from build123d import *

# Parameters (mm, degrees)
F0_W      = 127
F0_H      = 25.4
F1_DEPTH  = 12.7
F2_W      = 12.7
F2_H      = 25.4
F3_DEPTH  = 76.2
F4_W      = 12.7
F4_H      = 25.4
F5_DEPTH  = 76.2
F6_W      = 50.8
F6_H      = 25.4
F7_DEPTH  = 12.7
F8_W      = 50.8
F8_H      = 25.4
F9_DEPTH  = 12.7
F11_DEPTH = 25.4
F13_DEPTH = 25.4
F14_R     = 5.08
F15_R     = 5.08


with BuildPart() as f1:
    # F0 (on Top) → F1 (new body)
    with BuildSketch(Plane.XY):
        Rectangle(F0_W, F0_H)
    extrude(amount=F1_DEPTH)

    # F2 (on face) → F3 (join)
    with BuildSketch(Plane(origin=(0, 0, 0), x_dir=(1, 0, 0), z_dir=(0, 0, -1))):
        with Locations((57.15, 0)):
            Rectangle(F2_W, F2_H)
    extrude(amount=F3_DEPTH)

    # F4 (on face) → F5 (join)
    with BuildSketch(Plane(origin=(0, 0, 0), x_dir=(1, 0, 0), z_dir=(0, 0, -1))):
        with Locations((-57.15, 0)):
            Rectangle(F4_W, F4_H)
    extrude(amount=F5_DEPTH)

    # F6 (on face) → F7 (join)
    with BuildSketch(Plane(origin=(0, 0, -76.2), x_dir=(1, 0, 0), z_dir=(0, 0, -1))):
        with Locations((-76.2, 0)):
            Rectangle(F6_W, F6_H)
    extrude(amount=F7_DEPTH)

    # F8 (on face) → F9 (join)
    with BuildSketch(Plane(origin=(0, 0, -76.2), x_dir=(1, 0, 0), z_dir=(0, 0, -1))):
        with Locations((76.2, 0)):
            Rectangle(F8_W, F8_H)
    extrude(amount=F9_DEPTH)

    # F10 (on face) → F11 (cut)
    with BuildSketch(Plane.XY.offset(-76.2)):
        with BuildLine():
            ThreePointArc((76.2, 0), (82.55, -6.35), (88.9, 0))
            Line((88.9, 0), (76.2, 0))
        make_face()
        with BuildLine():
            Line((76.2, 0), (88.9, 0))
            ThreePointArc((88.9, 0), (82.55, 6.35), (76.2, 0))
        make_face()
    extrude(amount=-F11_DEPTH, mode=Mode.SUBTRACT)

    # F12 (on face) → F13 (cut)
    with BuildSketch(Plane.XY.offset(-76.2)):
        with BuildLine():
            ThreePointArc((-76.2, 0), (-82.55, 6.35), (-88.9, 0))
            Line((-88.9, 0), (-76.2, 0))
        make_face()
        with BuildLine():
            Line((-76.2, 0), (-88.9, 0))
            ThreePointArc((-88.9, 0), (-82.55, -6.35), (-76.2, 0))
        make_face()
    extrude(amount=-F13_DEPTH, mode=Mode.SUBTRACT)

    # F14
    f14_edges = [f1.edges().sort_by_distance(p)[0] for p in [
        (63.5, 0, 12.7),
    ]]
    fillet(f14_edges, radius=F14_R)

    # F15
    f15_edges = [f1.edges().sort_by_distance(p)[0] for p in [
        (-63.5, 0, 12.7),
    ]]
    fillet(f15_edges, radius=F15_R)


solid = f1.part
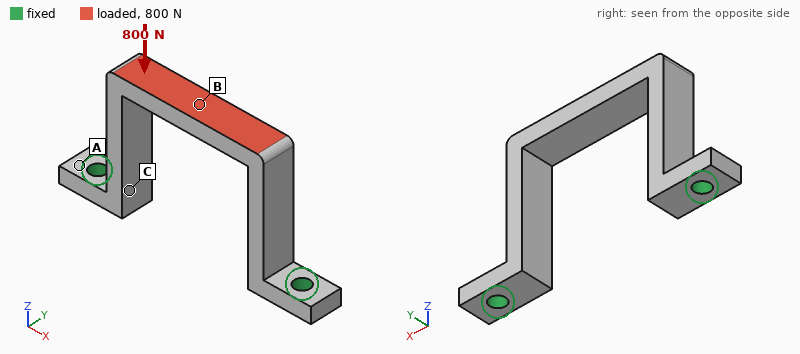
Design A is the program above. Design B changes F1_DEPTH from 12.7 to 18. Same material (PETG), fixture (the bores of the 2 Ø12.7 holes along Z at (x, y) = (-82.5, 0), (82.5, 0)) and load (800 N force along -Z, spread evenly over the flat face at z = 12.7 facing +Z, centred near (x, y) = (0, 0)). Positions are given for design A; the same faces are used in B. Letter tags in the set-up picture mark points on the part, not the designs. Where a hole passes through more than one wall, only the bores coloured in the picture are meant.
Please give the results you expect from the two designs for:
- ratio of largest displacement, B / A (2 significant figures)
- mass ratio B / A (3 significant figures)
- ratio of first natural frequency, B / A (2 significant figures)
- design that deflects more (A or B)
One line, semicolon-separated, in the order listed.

0.61; 1.14; 0.85; A
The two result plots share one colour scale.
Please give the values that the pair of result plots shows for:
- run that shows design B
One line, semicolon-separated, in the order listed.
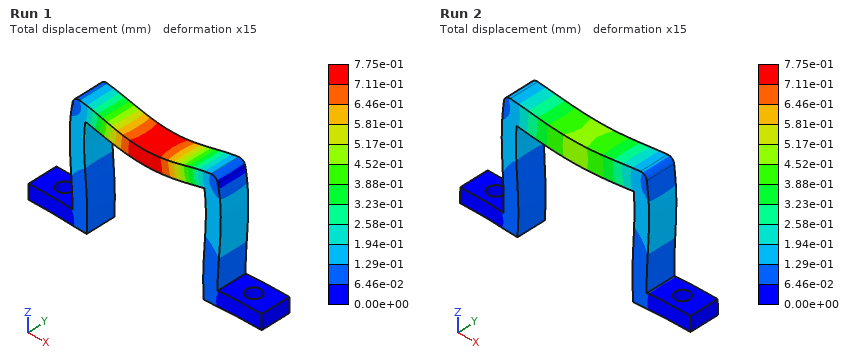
Run 2
